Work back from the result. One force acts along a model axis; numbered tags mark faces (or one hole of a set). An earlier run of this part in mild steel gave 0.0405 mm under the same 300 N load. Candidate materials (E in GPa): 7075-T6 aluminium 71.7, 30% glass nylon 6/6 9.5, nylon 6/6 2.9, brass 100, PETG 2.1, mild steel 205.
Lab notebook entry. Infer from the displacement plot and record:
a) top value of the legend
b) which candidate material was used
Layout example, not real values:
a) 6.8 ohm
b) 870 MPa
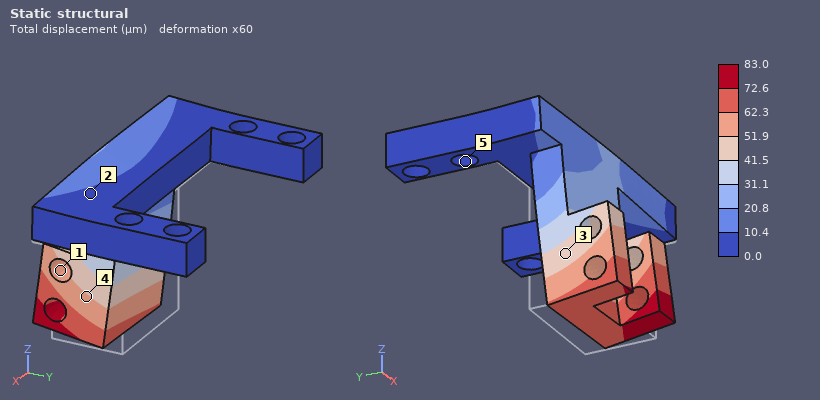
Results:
a) 83.0 µm
b) brass
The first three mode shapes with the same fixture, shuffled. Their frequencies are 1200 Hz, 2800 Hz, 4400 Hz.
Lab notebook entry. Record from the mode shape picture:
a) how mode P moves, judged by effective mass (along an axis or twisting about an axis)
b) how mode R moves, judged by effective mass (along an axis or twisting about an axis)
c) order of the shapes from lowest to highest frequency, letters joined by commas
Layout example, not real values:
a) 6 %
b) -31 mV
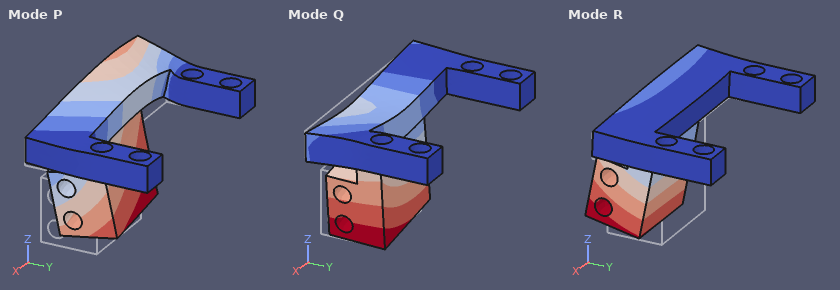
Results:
a) along Z
b) along Y
c) R, Q, P
